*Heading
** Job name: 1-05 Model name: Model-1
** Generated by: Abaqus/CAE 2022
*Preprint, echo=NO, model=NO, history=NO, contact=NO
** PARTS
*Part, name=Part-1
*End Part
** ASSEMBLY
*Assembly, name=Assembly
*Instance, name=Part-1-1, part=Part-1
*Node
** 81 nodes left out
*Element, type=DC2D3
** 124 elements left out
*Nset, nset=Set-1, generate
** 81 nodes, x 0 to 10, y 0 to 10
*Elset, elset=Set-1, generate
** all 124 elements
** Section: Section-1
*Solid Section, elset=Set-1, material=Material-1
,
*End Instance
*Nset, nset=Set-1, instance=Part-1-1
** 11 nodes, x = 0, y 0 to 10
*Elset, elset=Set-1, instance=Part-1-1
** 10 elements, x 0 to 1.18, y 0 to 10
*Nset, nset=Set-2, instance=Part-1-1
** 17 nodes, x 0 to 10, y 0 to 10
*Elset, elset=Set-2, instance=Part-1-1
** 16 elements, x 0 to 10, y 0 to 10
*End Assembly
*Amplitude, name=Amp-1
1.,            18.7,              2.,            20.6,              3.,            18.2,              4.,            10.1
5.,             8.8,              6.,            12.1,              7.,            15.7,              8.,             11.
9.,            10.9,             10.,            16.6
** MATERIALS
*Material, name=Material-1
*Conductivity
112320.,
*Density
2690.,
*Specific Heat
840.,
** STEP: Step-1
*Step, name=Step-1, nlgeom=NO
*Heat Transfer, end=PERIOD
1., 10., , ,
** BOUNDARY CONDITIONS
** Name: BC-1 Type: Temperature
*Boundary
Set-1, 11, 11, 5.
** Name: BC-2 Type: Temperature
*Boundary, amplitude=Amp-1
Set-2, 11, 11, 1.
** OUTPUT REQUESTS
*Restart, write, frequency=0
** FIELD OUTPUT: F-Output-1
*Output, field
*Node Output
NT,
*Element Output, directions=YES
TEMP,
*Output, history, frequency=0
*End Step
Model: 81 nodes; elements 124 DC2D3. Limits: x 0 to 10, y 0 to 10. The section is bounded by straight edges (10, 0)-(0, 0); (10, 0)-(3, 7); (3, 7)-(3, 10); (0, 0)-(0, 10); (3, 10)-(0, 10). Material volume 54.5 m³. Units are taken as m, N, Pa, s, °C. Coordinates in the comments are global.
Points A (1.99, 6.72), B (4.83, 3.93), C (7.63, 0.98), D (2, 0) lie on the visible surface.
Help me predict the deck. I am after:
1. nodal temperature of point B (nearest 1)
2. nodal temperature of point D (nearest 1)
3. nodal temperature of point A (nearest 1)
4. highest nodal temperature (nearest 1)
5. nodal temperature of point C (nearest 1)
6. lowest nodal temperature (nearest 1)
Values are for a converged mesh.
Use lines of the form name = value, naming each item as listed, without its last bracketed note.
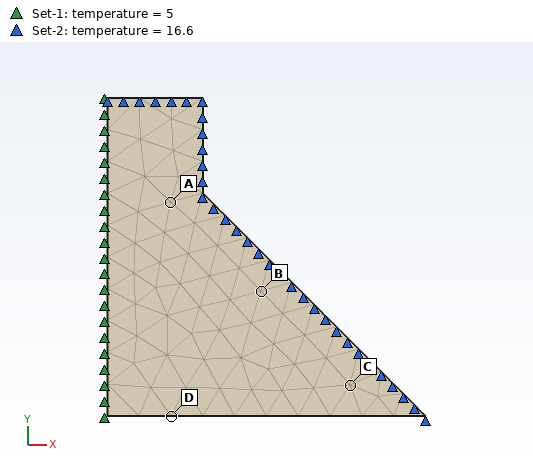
nodal temperature of point B = 5 °C
nodal temperature of point D = 0 °C
nodal temperature of point A = 3 °C
highest nodal temperature = 17 °C
nodal temperature of point C = 5 °C
lowest nodal temperature = 0 °C
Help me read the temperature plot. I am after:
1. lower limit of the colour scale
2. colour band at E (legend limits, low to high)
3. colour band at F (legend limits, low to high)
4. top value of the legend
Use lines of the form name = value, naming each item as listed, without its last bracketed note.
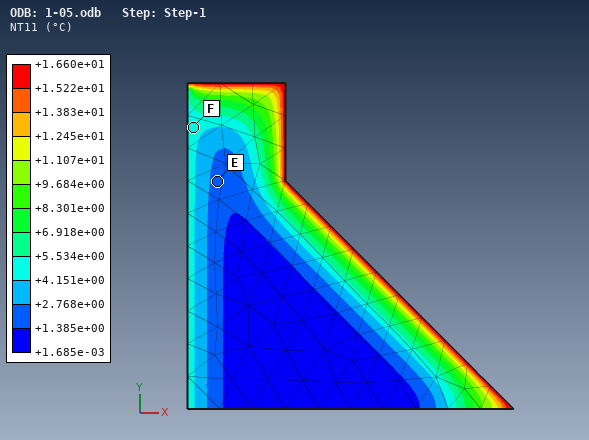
lower limit of the colour scale = +1.685e-03 °C
colour band at E = +1.385e+00 to +2.768e+00 °C
colour band at F = +4.151e+00 to +5.534e+00 °C
top value of the legend = +1.660e+01 °C
